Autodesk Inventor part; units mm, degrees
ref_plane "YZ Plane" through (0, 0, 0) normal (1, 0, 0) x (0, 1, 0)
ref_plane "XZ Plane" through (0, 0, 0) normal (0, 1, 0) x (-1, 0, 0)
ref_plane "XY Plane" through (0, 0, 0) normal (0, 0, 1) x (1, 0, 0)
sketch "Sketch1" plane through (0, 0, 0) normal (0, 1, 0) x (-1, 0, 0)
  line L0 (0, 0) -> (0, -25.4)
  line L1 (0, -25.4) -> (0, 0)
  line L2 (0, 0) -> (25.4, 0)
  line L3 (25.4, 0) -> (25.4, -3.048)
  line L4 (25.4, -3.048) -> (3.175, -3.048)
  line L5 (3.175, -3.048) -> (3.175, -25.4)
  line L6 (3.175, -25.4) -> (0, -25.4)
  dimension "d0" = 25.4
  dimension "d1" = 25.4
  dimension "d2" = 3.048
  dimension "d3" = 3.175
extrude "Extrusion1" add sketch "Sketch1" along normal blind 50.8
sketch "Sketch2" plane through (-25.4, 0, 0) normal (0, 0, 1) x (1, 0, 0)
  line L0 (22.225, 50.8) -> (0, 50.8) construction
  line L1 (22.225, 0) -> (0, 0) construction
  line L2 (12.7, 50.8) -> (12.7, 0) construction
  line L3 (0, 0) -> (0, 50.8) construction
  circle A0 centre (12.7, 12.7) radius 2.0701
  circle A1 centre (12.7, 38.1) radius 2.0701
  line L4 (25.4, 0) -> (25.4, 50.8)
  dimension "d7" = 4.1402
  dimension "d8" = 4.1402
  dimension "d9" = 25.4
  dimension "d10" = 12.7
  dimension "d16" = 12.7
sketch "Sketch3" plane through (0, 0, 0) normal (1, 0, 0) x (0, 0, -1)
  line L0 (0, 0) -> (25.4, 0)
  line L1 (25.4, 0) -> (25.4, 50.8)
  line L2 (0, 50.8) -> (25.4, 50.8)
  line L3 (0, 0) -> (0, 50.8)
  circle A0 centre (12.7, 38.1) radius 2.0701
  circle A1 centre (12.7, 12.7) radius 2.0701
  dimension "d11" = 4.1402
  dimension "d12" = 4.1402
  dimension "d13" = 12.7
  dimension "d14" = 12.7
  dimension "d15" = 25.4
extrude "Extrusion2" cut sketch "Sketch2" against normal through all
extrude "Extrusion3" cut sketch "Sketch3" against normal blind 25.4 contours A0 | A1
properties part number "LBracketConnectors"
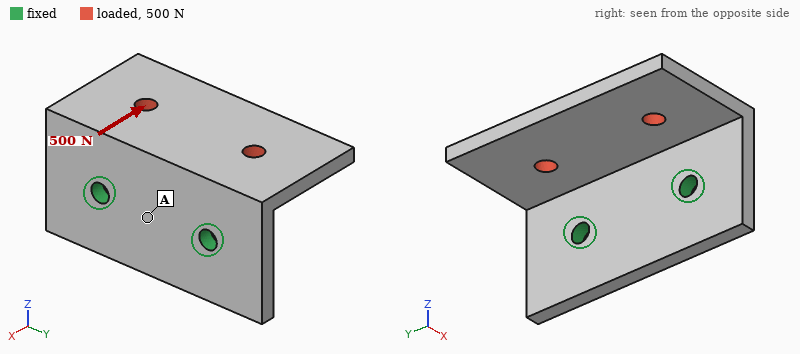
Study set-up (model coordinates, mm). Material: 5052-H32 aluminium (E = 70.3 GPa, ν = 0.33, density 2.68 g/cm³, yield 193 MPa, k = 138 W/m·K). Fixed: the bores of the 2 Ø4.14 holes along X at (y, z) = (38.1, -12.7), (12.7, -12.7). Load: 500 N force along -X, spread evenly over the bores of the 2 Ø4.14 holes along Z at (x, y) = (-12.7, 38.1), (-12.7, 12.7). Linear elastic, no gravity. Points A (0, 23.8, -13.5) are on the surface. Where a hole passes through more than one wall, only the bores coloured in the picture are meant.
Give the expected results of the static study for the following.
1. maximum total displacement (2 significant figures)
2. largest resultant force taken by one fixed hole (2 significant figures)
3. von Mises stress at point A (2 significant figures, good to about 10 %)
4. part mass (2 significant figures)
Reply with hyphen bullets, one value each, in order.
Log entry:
- 87 µm
- 250 N
- 16 MPa
- 20 g
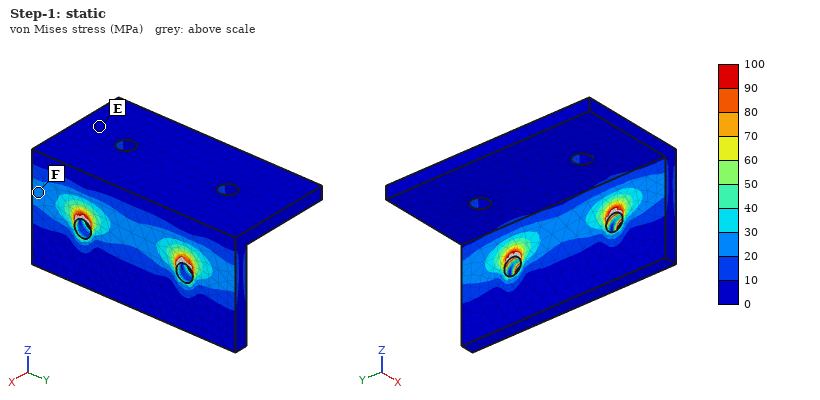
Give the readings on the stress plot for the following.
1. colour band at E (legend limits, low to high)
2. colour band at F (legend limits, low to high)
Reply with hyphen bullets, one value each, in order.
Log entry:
- 0 to 10 MPa
- 20 to 30 MPa
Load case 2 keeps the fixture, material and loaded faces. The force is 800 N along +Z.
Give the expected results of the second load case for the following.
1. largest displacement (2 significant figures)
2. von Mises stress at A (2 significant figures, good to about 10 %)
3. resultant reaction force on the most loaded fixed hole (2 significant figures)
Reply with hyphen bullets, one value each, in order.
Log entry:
- 0.34 mm
- 35 MPa
- 400 N
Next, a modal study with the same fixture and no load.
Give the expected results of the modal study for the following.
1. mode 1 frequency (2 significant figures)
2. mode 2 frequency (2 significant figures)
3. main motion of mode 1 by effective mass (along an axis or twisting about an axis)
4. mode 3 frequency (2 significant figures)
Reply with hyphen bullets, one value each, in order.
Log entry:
- 2700 Hz
- 4500 Hz
- along Z
- 7300 Hz
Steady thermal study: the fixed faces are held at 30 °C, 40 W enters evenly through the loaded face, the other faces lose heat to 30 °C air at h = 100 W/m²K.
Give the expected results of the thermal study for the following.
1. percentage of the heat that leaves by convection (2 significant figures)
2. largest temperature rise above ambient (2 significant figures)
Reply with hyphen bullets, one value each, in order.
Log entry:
- 25 %
- 43 K
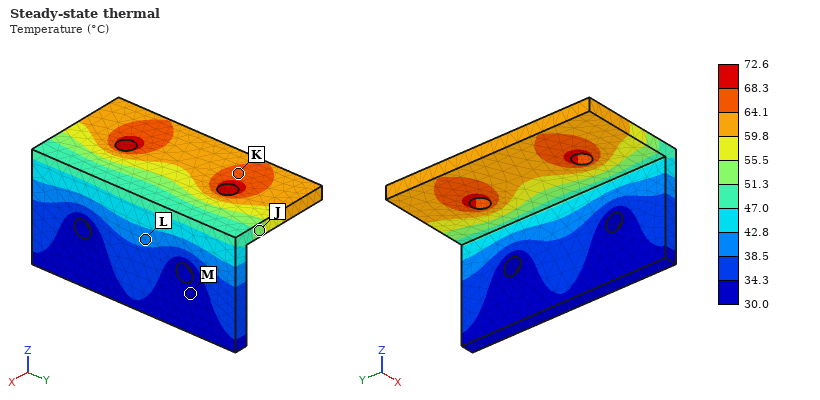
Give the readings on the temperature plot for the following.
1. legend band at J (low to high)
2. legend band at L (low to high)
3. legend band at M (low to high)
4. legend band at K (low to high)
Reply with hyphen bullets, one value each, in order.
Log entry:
- 51.3 to 55.5 °C
- 38.5 to 42.8 °C
- 30.0 to 34.3 °C
- 64.1 to 68.3 °C
